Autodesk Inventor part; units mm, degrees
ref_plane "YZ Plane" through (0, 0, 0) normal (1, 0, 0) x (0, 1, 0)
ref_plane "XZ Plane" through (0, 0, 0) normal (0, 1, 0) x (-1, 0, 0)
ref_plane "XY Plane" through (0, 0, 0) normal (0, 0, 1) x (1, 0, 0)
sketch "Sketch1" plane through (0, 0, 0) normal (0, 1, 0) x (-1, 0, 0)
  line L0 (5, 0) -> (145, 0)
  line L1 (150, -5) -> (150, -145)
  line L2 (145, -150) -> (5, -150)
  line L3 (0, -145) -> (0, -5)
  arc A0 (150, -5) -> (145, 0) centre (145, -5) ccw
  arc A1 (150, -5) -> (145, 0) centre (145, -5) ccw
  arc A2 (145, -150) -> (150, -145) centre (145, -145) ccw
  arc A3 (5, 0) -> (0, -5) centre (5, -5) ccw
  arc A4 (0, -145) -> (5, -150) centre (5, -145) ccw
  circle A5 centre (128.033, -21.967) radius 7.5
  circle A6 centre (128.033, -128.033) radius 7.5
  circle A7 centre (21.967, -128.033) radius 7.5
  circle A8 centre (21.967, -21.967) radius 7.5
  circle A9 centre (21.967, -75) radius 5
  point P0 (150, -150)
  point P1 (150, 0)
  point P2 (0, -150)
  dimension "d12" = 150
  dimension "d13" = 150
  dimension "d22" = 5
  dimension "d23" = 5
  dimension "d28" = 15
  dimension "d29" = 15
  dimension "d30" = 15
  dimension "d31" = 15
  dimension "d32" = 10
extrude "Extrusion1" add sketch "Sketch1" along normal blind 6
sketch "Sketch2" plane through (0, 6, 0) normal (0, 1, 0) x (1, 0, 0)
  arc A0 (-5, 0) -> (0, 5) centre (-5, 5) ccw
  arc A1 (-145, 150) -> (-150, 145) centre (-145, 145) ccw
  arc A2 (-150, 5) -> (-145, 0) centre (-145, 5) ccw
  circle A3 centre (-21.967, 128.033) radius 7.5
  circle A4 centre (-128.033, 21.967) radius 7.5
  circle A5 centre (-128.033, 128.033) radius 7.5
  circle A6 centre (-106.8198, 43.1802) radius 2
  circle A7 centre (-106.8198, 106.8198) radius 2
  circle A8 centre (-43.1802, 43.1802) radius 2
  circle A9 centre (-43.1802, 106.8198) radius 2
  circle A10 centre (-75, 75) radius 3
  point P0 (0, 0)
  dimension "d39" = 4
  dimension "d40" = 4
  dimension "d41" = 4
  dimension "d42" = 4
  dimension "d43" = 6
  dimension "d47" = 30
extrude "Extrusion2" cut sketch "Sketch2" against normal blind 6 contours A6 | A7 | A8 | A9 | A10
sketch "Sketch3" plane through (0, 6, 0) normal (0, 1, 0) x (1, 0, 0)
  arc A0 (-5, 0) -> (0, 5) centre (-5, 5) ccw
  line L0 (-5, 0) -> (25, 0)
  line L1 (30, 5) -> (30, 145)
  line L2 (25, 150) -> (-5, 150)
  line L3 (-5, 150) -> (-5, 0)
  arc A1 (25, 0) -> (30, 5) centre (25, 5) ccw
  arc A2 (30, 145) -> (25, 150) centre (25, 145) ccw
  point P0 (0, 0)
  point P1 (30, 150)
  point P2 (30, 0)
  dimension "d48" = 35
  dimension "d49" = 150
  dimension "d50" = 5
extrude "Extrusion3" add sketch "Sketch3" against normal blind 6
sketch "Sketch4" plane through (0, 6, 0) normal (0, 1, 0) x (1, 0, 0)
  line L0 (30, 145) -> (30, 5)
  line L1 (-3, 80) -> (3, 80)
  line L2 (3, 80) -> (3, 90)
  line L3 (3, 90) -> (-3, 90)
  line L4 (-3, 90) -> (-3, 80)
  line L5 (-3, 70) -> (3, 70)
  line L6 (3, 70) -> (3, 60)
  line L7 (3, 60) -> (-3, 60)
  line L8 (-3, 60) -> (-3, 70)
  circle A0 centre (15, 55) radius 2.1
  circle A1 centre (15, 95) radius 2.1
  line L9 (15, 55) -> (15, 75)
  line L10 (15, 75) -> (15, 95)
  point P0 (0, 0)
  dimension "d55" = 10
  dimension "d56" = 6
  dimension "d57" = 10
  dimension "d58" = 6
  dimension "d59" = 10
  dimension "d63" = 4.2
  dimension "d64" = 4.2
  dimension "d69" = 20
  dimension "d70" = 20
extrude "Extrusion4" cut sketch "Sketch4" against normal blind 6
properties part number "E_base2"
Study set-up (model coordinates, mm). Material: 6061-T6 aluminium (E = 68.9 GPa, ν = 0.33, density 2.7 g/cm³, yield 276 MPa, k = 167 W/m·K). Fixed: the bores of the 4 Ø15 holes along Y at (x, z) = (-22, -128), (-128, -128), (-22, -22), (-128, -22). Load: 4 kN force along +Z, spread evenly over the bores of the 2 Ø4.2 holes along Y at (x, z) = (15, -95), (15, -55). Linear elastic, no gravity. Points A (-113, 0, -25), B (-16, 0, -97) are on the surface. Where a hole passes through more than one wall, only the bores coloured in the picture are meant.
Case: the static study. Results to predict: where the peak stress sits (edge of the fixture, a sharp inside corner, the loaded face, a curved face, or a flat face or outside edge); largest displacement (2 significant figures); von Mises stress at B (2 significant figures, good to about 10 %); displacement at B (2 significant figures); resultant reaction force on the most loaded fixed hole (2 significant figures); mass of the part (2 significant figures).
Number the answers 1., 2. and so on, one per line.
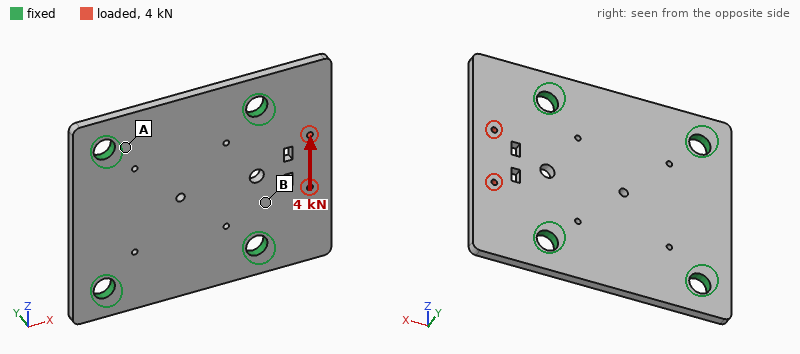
1. the loaded face
2. 13 µm
3. 6.6 MPa
4. 2.8 µm
5. 2.3 kN
6. 420 g
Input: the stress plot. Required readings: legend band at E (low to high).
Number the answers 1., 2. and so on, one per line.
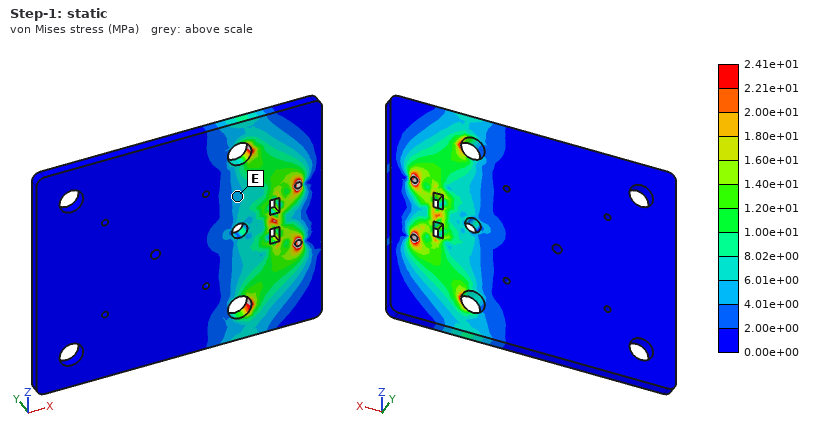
1. 4.01e+00 to 6.01e+00 MPa
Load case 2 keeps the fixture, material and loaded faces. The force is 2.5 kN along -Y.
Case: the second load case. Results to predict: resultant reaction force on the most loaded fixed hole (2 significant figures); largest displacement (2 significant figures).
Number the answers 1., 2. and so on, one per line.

1. 1.3 kN
2. 0.64 mm
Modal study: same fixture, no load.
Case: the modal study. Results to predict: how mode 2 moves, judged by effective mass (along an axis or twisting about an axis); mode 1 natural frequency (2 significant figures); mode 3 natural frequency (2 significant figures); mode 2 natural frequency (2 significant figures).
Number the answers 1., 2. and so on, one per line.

1. along Y
2. 1700 Hz
3. 2600 Hz
4. 2300 Hz
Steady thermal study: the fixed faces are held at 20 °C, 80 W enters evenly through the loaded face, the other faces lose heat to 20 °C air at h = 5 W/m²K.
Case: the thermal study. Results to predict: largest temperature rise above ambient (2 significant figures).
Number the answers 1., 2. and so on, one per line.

1. 44 K
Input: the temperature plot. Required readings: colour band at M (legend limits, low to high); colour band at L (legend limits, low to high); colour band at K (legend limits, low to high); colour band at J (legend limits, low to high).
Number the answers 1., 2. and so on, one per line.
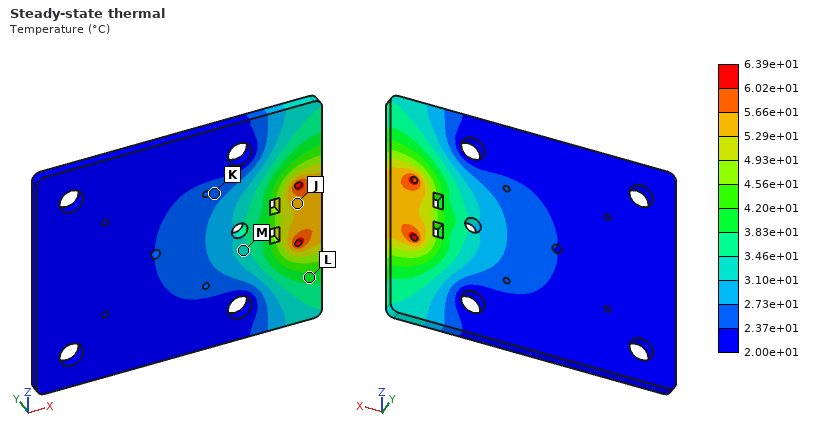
1. 3.10e+01 to 3.46e+01 °C
2. 3.83e+01 to 4.20e+01 °C
3. 2.37e+01 to 2.73e+01 °C
4. 5.29e+01 to 5.66e+01 °C
